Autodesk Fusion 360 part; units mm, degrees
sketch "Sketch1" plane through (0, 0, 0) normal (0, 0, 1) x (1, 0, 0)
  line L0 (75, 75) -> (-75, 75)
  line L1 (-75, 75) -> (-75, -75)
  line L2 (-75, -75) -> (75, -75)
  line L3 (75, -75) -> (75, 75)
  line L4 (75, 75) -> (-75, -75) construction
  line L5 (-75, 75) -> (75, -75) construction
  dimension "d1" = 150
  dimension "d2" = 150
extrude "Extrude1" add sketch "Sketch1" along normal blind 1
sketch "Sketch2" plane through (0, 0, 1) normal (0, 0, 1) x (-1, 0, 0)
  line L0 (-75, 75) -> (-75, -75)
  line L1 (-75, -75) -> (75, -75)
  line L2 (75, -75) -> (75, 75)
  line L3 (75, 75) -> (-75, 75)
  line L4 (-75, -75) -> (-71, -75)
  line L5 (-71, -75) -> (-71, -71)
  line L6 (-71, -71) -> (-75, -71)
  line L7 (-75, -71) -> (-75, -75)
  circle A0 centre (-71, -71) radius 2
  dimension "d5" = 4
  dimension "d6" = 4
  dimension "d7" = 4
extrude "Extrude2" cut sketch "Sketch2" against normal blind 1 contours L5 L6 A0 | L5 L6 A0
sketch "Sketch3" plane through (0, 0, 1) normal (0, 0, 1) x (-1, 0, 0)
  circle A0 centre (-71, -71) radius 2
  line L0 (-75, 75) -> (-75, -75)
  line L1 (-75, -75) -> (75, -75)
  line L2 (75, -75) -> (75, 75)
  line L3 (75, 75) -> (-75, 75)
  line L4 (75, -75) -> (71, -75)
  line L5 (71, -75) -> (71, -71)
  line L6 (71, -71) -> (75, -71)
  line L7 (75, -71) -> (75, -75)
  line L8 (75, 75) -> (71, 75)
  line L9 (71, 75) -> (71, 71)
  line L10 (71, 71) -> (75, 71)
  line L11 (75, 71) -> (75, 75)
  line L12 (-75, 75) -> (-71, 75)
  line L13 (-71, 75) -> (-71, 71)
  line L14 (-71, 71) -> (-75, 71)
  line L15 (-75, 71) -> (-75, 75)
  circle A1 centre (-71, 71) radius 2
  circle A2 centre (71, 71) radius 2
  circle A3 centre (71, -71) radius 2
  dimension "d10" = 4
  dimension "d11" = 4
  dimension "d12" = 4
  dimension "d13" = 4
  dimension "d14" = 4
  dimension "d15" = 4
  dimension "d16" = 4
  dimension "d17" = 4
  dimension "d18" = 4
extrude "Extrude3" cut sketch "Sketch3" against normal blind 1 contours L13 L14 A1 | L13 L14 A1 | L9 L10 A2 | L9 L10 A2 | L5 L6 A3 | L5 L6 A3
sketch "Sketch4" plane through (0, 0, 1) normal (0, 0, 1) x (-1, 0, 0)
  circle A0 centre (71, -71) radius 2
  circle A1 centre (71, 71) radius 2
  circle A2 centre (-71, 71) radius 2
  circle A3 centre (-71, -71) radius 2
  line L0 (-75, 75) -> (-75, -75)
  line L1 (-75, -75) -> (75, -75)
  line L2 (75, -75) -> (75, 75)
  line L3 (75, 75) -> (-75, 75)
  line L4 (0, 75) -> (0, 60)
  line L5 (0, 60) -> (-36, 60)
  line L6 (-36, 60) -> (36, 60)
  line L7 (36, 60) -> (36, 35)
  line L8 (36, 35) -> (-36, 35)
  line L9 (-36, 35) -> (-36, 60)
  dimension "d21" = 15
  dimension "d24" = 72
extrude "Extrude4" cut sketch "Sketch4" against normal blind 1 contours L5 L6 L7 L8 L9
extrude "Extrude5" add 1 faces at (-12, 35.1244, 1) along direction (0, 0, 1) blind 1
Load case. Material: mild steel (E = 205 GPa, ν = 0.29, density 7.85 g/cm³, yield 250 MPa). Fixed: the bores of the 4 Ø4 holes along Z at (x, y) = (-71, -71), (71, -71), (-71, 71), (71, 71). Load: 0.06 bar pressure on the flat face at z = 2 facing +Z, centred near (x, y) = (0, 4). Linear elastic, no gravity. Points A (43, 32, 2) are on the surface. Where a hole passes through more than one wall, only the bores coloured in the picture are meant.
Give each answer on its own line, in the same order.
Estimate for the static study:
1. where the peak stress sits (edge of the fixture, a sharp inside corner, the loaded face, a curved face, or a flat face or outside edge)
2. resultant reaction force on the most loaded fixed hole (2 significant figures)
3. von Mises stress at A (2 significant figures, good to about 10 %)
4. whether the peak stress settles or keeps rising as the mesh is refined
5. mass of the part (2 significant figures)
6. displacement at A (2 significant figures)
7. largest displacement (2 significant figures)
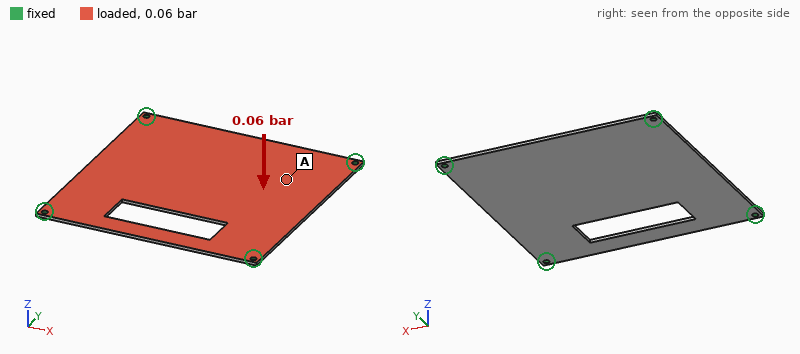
edge of the fixture
33 N
7.1 MPa
keeps rising
320 g
0.100 mm
0.16 mm
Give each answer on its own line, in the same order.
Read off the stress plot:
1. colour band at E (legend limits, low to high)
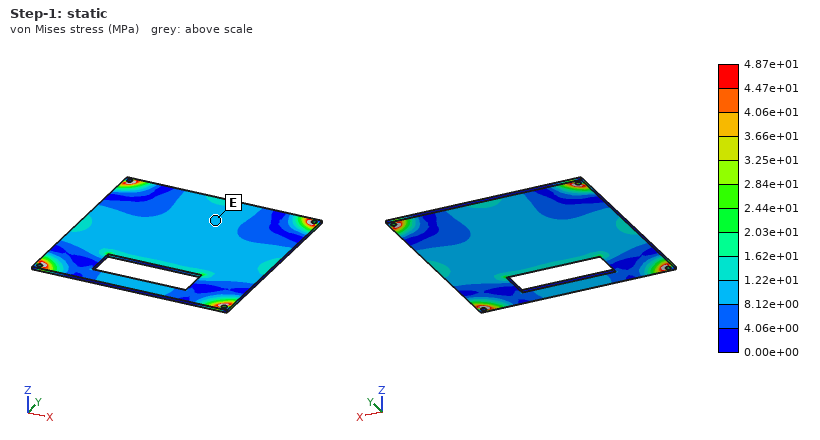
8.12e+00 to 1.22e+01 MPa
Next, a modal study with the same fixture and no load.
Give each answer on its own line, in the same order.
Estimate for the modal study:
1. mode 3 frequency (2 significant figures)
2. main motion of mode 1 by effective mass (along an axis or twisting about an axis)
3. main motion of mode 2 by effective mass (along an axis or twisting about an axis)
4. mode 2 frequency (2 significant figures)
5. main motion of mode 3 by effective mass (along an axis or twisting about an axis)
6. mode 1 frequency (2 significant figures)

570 Hz
along Z
twisting about Y
540 Hz
twisting about X
290 Hz
